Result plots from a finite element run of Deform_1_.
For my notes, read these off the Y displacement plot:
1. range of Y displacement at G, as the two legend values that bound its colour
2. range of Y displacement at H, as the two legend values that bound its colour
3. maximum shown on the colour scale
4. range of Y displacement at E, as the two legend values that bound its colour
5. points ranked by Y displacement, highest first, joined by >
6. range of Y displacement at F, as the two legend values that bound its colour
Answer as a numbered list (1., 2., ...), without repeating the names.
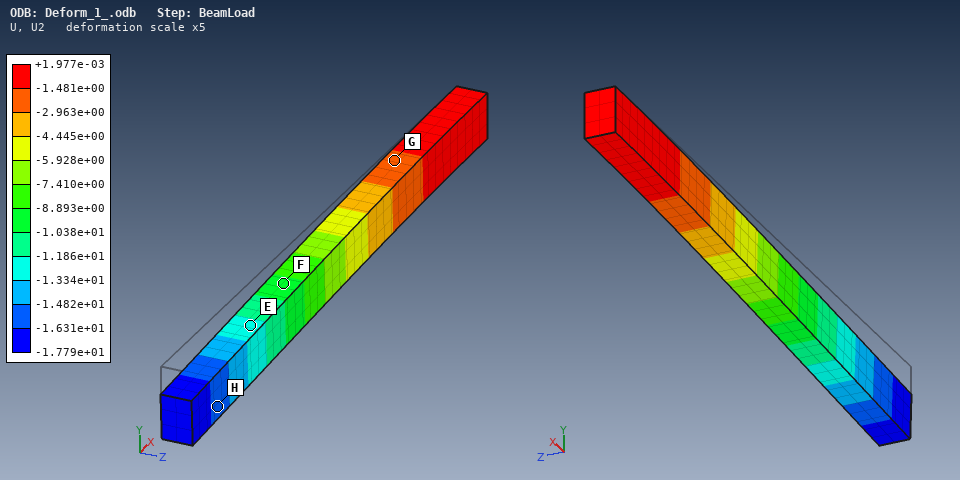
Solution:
1. -2.963e+00 to -1.481e+00
2. -1.631e+01 to -1.482e+01
3. +1.977e-03
4. -1.334e+01 to -1.186e+01
5. G > F > E > H
6. -1.038e+01 to -8.893e+00
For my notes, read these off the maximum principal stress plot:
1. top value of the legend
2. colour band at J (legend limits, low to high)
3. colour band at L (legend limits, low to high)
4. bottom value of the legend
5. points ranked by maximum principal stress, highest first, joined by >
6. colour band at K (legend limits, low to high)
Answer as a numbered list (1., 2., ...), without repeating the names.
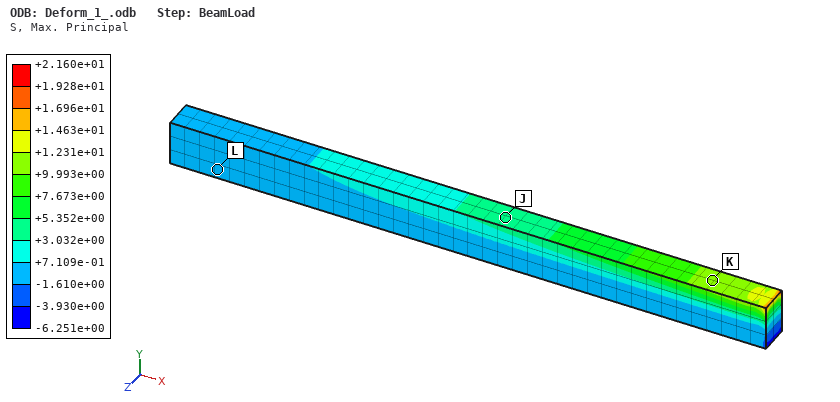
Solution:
1. +2.160e+01
2. +3.032e+00 to +5.352e+00
3. -1.610e+00 to +7.109e-01
4. -6.251e+00
5. K > J > L
6. +9.993e+00 to +1.231e+01
